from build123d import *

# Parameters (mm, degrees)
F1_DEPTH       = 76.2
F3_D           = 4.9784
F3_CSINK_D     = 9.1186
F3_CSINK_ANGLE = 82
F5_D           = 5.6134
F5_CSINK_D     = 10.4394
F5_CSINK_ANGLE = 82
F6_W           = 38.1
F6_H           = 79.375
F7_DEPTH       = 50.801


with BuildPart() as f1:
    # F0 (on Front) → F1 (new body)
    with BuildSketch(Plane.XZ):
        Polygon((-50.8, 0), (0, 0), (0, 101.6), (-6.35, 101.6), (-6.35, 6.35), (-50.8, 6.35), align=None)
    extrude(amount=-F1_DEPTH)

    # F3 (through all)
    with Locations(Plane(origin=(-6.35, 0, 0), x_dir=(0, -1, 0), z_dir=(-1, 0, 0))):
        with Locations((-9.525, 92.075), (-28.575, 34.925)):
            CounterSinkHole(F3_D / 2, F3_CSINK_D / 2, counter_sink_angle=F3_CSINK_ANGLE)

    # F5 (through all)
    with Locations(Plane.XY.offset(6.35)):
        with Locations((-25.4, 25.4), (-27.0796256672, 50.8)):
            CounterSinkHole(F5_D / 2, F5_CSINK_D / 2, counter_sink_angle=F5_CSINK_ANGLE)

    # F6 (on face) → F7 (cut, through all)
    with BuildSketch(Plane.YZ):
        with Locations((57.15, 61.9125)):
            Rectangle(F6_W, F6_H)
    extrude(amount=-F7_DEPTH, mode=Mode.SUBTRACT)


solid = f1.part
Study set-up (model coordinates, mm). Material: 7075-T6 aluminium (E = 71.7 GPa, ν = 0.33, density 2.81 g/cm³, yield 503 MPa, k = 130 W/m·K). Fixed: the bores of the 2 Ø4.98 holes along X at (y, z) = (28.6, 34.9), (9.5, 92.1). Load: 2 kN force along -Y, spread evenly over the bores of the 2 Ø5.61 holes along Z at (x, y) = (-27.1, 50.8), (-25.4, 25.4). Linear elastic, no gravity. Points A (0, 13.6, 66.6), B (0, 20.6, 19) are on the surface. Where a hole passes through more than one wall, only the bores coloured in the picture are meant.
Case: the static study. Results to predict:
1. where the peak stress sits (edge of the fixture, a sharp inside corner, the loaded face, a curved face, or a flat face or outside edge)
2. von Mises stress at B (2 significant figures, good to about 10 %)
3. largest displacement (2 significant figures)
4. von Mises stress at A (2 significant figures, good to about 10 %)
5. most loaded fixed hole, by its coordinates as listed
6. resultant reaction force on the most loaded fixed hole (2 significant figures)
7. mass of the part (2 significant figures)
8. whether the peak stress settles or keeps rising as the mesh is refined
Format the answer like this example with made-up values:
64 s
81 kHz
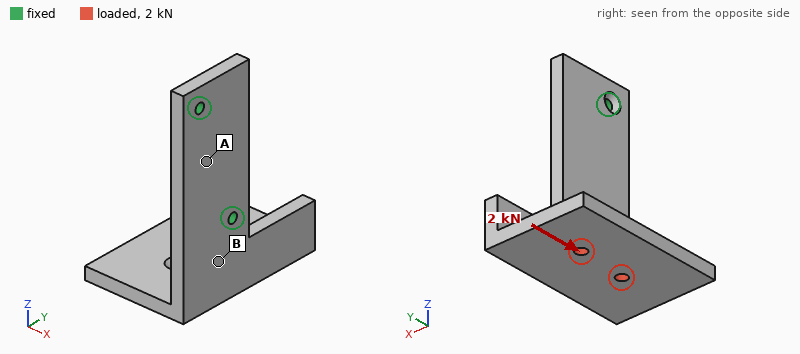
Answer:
edge of the fixture
95 MPa
1.4 mm
48 MPa
(28.6, 34.9)
2.9 kN
140 g
keeps rising
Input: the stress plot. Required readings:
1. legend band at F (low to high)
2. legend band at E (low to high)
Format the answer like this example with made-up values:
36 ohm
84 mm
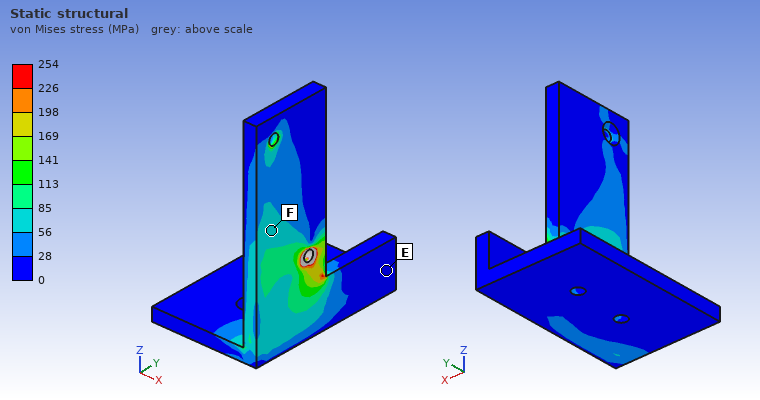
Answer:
56 to 85 MPa
0 to 28 MPa
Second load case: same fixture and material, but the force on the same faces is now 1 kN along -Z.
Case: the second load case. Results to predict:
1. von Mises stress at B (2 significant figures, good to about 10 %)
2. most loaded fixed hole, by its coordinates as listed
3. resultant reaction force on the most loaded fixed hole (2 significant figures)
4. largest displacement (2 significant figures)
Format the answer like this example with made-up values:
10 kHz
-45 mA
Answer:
72 MPa
(28.6, 34.9)
720 N
0.87 mm
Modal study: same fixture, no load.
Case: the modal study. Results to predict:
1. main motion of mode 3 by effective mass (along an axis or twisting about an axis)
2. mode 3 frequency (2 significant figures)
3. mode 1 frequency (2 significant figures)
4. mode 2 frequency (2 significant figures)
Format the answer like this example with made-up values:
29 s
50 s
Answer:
along X
2200 Hz
660 Hz
820 Hz
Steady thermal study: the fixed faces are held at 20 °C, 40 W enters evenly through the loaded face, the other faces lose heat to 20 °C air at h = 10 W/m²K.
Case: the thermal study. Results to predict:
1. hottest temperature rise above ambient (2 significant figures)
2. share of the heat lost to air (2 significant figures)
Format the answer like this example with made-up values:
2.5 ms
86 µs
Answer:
63 K
15 %
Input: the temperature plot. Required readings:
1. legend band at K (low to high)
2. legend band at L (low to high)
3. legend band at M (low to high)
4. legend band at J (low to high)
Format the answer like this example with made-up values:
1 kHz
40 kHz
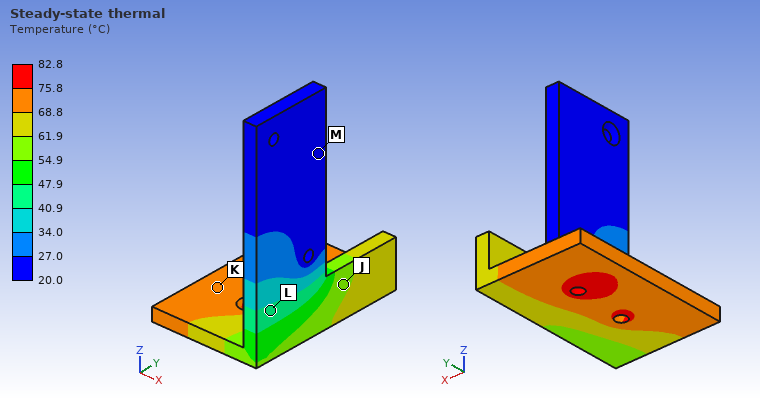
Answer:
68.8 to 75.8 °C
40.9 to 47.9 °C
20.0 to 27.0 °C
54.9 to 61.9 °C
